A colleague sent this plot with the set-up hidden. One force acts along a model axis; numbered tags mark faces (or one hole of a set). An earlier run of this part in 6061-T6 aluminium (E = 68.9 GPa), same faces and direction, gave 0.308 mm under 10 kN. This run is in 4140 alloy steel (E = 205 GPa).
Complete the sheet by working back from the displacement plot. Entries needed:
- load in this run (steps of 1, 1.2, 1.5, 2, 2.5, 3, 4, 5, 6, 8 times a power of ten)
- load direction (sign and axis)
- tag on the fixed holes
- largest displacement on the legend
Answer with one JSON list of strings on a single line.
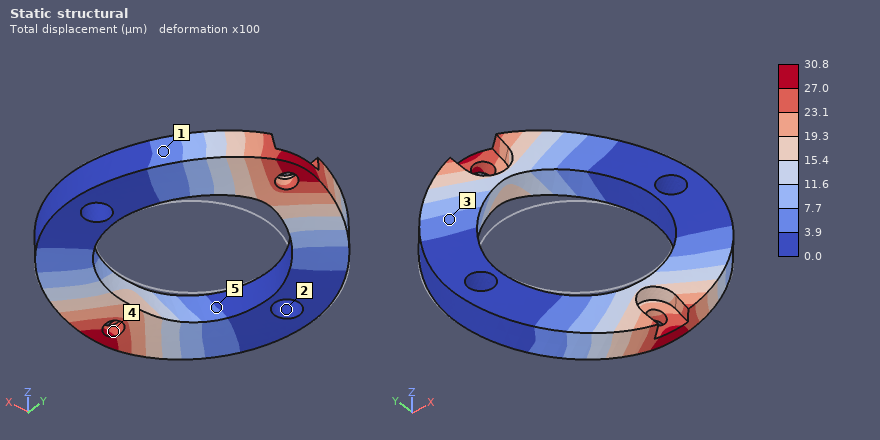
["3 kN", "+Y", "2", "30.8 µm"]
